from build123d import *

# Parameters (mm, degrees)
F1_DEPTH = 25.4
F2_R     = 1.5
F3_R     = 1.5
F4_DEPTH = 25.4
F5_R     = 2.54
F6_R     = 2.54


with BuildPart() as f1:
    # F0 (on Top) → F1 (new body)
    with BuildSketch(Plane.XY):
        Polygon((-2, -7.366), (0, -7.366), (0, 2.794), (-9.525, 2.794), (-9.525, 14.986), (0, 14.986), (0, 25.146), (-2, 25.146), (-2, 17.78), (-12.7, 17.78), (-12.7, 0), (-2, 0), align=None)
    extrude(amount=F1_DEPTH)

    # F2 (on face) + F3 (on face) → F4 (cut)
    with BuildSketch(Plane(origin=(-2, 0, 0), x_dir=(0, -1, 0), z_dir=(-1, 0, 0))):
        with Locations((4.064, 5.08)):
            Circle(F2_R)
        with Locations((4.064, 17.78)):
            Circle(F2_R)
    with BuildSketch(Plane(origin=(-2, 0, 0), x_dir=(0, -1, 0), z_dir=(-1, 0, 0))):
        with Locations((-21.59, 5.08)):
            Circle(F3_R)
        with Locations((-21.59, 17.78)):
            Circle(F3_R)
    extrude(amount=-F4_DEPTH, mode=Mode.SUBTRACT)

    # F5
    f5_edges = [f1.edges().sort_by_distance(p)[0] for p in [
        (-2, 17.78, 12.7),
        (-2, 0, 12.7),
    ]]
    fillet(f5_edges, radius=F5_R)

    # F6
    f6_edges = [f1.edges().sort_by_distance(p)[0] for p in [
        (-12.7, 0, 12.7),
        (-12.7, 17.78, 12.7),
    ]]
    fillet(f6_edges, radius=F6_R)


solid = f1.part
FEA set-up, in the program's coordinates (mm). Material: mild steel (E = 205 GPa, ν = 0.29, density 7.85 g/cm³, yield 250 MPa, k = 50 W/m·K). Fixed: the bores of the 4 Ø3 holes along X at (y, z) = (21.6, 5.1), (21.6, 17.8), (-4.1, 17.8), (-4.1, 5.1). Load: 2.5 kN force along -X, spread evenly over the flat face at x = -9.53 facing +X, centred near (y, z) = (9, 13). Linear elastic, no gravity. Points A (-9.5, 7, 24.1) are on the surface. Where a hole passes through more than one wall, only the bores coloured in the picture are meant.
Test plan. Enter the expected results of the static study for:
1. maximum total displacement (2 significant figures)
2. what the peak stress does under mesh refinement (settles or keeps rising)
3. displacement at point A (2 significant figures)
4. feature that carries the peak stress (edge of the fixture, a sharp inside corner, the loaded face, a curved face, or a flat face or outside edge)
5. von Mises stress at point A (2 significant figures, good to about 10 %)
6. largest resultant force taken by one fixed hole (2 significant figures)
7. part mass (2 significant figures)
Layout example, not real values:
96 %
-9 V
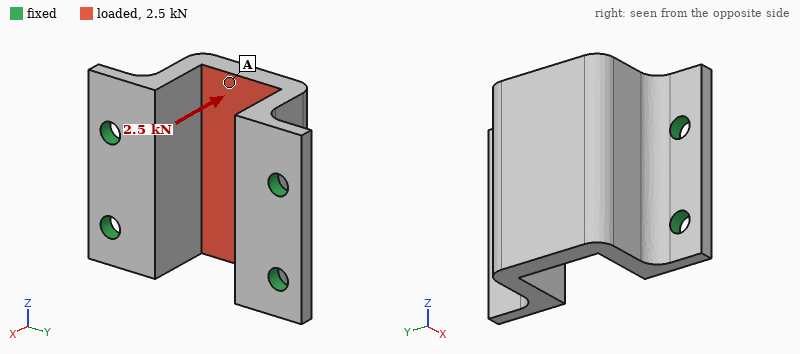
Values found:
9.7 µm
keeps rising
9.0 µm
edge of the fixture
32 MPa
850 N
27 g
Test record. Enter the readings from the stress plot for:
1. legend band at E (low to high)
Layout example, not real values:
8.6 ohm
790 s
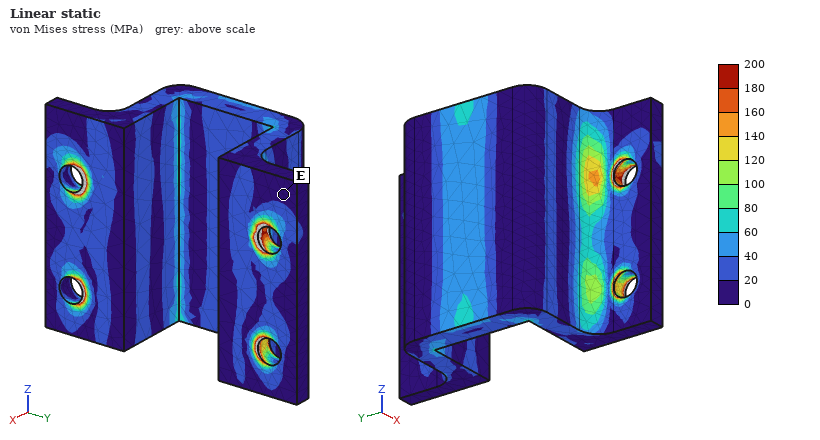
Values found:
0 to 20 MPa
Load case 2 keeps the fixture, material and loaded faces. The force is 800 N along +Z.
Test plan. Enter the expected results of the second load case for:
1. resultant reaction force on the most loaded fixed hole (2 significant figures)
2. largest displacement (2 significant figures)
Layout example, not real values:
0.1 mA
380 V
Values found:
370 N
5.8 µm
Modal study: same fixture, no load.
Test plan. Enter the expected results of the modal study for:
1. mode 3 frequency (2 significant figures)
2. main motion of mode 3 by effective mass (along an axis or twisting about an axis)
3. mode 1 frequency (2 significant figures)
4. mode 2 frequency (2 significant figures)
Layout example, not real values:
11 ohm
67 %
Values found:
18 kHz
twisting about X
15 kHz
15 kHz
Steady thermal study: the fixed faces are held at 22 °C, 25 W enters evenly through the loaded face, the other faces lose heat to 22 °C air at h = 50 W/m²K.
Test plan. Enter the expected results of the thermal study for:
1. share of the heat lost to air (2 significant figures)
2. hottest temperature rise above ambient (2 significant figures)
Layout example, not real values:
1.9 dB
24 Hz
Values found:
14 %
58 K
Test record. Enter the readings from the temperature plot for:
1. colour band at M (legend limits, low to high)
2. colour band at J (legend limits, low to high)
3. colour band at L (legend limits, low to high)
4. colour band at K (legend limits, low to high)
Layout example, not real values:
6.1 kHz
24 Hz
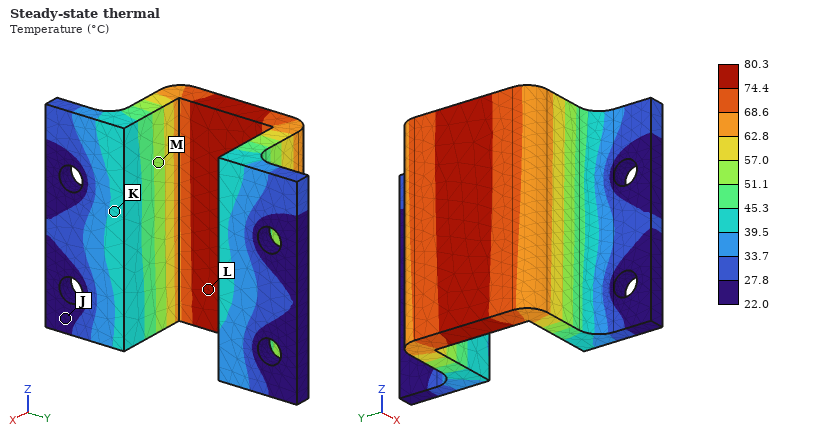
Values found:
51.1 to 57.0 °C
22.0 to 27.8 °C
74.4 to 80.3 °C
39.5 to 45.3 °C
